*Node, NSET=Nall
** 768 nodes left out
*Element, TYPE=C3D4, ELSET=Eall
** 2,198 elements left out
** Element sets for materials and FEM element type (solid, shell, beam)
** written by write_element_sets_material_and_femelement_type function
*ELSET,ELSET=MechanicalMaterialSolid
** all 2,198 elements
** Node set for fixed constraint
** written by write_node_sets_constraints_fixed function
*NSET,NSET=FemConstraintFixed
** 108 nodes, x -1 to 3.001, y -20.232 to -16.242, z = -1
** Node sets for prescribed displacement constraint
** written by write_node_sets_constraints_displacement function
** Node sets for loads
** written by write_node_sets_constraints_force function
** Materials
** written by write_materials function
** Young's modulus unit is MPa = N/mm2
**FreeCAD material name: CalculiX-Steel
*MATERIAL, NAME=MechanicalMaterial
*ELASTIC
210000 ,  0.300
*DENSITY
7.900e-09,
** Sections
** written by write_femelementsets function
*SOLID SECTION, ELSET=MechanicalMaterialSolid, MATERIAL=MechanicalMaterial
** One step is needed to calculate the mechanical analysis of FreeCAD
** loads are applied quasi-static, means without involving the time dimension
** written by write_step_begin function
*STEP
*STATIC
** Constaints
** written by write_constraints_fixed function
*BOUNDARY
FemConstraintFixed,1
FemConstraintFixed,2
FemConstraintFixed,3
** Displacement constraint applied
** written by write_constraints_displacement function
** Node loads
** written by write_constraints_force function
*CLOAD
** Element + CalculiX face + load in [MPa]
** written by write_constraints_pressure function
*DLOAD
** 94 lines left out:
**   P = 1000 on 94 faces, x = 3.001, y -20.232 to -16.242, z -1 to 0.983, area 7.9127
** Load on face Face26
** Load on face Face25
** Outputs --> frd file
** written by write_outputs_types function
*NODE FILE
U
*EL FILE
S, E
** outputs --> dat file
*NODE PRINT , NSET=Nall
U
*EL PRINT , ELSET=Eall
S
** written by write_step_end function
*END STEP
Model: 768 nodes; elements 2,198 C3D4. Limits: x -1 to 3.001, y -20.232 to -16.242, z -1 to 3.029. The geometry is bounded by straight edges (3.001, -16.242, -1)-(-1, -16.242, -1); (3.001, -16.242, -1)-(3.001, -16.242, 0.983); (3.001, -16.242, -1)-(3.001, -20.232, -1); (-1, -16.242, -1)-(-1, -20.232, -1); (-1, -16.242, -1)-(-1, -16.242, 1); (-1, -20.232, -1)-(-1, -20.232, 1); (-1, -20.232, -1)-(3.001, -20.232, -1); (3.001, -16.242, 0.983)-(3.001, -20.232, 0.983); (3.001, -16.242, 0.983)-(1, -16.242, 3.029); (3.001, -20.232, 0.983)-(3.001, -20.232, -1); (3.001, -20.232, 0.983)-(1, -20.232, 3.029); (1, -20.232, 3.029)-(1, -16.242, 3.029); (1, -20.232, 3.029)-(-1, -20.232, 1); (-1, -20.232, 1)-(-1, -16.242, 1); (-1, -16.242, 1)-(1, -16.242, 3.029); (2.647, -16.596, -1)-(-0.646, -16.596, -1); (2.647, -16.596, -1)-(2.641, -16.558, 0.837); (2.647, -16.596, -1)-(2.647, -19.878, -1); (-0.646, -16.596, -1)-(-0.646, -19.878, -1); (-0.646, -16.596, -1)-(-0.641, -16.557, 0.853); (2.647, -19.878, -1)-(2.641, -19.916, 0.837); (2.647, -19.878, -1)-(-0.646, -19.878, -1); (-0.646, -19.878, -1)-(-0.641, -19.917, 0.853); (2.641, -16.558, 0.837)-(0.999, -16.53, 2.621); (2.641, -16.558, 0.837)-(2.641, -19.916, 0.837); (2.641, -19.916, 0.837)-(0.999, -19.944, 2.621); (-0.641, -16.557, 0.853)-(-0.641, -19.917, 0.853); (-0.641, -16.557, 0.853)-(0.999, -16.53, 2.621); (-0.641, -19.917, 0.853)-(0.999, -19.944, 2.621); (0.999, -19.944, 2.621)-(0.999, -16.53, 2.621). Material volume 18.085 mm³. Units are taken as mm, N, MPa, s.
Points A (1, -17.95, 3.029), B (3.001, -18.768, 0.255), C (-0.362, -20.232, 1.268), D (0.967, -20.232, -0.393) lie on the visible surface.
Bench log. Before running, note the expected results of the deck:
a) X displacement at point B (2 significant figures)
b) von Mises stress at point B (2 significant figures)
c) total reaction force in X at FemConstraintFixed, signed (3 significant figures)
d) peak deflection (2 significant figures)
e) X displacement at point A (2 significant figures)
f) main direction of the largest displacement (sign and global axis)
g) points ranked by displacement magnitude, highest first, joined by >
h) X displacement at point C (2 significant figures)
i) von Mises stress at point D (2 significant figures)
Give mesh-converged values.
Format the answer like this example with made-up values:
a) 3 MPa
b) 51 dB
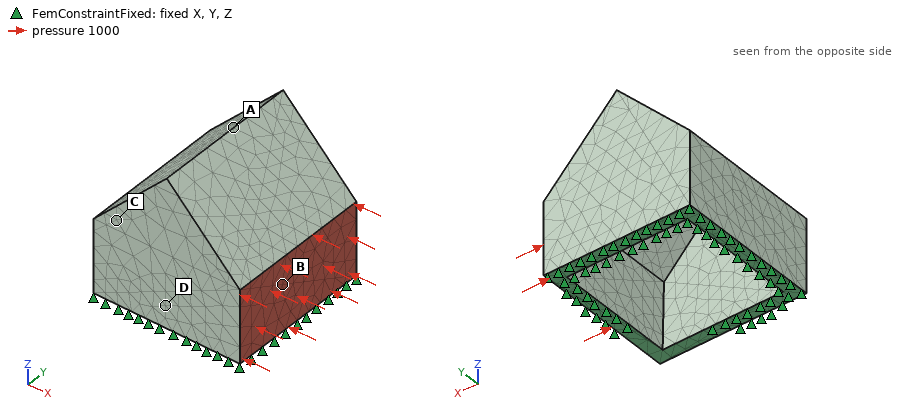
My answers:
a) -0.15 mm
b) 8500 MPa
c) 7910 N
d) 0.17 mm
e) -0.079 mm
f) -X
g) B > A > C > D
h) -0.038 mm
i) 3100 MPa
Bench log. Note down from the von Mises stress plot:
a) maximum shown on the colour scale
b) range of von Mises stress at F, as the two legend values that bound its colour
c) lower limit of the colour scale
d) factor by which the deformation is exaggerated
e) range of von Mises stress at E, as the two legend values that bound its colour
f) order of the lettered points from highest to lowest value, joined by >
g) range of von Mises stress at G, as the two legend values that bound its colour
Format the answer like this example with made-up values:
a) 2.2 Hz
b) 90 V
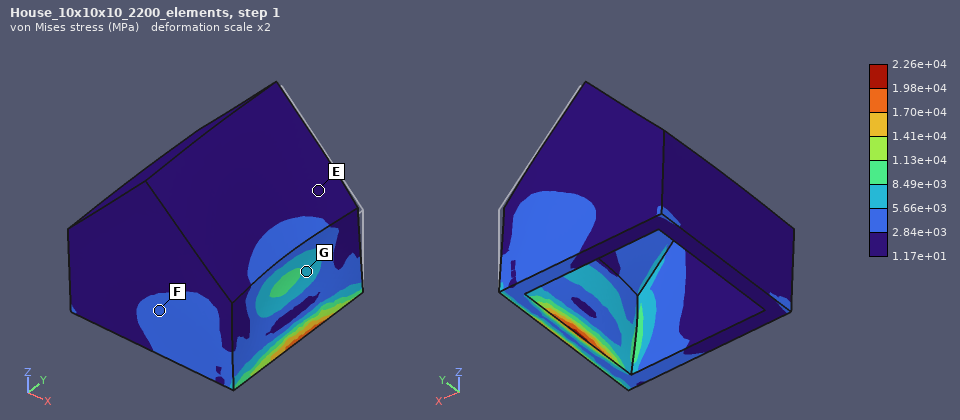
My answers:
a) 2.26e+04 MPa
b) 2.84e+03 to 5.66e+03 MPa
c) 1.17e+01 MPa
d) 2
e) 1.17e+01 to 2.84e+03 MPa
f) G > F > E
g) 5.66e+03 to 8.49e+03 MPa
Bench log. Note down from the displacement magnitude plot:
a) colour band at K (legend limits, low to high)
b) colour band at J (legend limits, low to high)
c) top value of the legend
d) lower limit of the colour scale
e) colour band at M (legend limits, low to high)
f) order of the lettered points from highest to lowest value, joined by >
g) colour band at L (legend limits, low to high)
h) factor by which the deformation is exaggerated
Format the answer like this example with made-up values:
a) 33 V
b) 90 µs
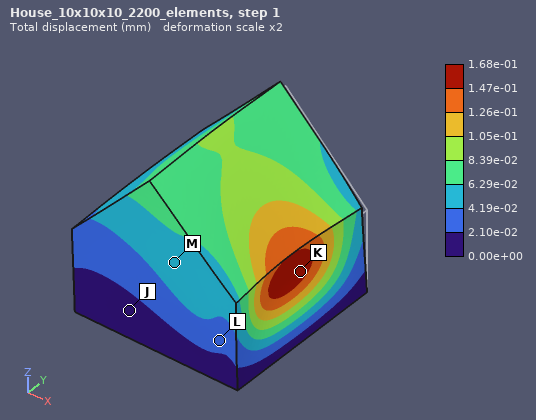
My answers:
a) 1.47e-01 to 1.68e-01 mm
b) 0.00e+00 to 2.10e-02 mm
c) 1.68e-01 mm
d) 0.00e+00 mm
e) 4.19e-02 to 6.29e-02 mm
f) K > M > L > J
g) 2.10e-02 to 4.19e-02 mm
h) 2
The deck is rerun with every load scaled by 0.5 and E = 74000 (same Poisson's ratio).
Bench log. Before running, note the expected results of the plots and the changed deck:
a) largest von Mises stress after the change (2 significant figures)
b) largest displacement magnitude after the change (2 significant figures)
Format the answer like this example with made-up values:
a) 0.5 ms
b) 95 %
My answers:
a) 11000 MPa
b) 0.24 mm
